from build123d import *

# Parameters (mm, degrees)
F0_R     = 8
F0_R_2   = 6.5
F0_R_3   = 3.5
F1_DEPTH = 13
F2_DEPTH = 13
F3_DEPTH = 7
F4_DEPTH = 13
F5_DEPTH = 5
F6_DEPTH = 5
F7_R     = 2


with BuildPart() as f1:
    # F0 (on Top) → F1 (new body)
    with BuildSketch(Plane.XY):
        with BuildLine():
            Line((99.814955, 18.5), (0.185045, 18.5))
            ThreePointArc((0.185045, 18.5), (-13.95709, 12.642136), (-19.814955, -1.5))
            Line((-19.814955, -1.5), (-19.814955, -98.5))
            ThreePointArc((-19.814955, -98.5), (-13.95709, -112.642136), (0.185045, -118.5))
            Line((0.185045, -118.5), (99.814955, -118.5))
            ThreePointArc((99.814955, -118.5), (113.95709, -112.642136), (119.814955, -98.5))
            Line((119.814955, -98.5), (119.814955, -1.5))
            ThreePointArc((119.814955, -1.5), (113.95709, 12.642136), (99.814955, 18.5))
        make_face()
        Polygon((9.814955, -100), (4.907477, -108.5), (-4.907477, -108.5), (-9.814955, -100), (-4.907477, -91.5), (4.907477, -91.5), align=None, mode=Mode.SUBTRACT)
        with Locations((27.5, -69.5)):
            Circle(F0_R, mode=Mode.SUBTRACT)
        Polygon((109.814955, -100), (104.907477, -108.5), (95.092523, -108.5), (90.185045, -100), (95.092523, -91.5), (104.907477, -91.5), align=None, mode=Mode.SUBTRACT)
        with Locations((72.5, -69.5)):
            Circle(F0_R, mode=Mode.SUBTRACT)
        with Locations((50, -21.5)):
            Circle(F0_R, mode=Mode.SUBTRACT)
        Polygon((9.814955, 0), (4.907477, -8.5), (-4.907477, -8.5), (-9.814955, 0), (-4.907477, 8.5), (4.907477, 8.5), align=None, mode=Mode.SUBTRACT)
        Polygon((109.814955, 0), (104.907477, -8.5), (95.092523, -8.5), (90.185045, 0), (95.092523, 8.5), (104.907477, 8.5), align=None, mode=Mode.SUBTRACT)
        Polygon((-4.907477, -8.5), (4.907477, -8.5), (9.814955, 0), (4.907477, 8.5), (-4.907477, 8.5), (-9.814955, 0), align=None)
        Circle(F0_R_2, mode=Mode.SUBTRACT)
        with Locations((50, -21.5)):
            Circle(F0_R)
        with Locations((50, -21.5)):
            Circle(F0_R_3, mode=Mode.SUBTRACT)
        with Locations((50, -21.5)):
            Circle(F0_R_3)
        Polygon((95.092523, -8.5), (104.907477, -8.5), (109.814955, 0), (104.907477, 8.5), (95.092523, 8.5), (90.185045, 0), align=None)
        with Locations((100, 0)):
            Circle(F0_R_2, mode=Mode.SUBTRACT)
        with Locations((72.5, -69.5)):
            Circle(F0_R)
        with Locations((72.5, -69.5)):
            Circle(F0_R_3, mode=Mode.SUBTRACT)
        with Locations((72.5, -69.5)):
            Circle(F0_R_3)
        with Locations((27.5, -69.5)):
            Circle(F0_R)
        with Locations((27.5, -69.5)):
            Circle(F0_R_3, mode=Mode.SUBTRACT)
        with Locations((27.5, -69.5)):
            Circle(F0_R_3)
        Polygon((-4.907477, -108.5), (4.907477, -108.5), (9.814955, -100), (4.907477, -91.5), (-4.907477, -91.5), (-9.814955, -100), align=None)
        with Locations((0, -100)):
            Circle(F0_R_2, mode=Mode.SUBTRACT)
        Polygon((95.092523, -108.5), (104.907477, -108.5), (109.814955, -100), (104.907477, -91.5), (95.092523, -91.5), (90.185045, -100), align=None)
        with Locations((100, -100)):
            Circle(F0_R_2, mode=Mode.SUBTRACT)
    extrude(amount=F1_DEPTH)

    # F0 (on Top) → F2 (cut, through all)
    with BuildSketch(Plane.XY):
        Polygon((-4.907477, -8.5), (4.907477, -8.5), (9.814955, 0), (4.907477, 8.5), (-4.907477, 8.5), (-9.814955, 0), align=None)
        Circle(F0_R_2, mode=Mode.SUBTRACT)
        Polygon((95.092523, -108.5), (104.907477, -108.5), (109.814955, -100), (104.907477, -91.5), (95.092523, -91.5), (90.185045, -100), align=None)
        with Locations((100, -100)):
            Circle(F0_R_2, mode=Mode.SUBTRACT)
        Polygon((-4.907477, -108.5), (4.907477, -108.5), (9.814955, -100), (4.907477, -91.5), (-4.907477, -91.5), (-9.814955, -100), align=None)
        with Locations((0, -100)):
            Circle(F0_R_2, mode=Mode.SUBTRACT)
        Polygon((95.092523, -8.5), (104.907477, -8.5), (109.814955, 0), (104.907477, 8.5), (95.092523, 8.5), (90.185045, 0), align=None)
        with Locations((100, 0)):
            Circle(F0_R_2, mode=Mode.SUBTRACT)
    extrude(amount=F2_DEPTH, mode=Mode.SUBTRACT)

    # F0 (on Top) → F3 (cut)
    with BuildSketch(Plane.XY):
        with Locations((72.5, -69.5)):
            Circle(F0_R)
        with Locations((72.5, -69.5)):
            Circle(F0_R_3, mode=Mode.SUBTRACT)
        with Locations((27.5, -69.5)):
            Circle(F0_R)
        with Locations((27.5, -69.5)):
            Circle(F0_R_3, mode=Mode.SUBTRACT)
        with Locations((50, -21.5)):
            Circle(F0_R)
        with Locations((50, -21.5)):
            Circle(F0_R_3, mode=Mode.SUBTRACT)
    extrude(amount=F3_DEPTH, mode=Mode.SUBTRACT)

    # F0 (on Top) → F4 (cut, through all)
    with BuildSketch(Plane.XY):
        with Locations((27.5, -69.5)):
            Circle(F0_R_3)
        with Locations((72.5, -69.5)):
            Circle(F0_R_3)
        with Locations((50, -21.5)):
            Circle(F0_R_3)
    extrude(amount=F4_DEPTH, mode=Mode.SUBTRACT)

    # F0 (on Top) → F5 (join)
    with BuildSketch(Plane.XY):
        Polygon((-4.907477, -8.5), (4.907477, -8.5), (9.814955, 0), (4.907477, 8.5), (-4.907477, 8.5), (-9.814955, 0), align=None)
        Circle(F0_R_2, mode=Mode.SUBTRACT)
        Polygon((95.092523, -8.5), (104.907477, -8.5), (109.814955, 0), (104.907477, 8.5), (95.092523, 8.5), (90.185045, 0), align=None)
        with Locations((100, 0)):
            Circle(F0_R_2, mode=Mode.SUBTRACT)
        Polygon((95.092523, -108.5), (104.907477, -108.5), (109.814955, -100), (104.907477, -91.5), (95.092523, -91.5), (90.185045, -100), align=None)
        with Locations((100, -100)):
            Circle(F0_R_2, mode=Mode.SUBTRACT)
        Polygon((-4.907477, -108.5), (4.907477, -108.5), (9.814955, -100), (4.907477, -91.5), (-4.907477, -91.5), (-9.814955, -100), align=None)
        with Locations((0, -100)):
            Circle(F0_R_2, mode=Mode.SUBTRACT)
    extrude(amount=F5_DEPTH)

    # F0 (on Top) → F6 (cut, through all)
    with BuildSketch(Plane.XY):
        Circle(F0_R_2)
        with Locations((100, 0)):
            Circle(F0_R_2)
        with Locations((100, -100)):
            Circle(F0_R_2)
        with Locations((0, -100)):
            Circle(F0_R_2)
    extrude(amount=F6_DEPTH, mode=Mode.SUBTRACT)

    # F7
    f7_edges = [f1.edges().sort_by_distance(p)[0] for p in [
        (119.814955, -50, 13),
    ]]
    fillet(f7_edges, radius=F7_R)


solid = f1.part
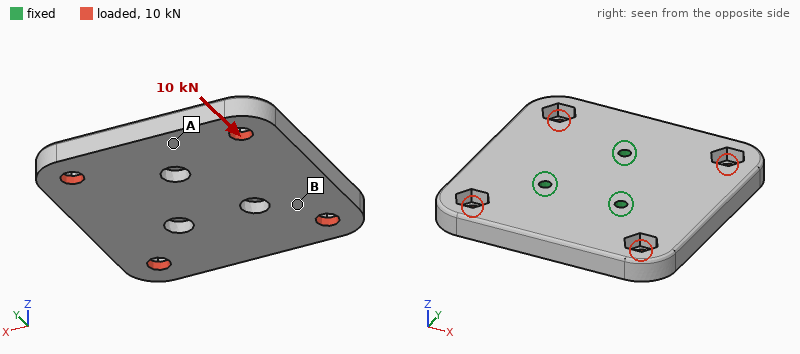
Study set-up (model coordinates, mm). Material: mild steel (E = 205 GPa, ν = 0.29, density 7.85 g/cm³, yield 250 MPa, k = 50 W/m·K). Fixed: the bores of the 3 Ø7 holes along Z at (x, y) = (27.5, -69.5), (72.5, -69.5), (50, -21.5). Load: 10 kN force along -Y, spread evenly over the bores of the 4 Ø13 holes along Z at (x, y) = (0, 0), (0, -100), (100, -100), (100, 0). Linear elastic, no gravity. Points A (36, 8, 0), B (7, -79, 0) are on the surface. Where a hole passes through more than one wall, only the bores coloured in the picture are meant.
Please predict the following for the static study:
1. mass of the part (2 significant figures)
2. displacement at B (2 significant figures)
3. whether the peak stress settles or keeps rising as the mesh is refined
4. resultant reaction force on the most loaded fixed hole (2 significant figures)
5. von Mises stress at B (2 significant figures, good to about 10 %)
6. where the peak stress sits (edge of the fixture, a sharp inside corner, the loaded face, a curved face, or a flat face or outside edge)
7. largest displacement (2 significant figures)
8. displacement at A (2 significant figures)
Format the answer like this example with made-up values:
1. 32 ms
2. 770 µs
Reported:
1. 1.8 kg
2. 4.0 µm
3. keeps rising
4. 3.5 kN
5. 11 MPa
6. edge of the fixture
7. 14 µm
8. 5.9 µm
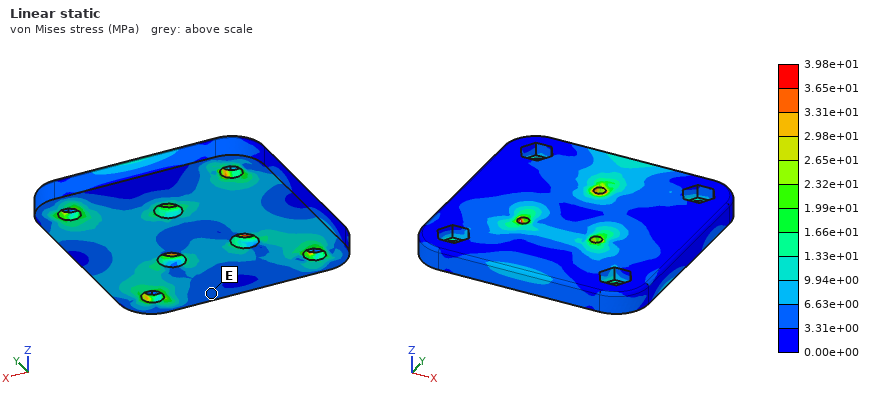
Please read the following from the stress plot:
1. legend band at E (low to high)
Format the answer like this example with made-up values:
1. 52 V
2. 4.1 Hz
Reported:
1. 3.31e+00 to 6.63e+00 MPa
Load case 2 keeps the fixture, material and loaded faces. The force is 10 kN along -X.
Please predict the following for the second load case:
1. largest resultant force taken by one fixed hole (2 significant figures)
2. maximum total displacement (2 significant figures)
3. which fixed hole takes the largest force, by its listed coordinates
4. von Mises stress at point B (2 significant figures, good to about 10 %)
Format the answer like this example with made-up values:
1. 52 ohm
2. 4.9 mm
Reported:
1. 3.9 kN
2. 21 µm
3. (50, -21.5)
4. 6.0 MPa
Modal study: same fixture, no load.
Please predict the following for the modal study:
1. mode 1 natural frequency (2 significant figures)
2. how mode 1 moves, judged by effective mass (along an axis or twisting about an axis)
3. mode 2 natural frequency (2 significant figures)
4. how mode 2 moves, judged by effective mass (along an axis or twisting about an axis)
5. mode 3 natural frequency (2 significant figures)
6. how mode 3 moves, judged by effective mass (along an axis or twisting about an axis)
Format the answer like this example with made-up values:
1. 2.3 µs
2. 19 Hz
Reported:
1. 1900 Hz
2. twisting about Y
3. 2300 Hz
4. along Z
5. 2900 Hz
6. along Z
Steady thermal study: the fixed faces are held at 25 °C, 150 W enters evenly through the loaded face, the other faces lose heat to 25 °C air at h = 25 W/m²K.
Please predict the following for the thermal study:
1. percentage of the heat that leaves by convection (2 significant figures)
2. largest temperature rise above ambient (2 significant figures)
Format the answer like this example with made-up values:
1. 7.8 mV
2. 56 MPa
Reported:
1. 30 %
2. 79 K
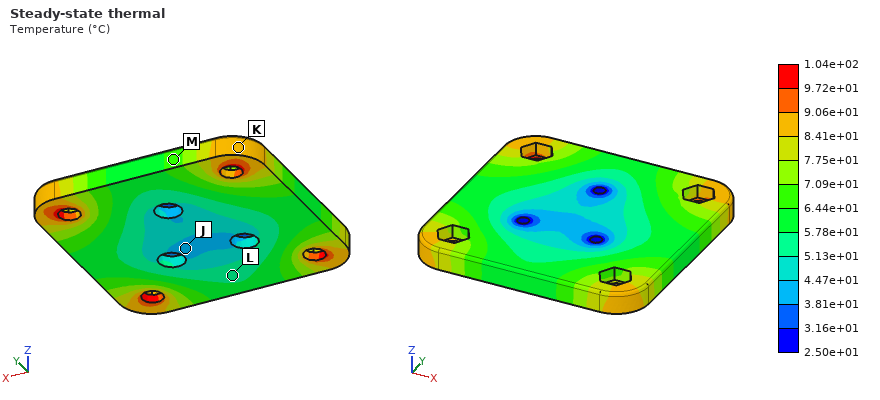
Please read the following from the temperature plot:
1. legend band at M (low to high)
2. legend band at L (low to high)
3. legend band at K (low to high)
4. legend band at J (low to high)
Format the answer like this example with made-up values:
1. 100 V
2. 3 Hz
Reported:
1. 6.44e+01 to 7.09e+01 °C
2. 5.13e+01 to 5.78e+01 °C
3. 8.41e+01 to 9.06e+01 °C
4. 3.81e+01 to 4.47e+01 °C
